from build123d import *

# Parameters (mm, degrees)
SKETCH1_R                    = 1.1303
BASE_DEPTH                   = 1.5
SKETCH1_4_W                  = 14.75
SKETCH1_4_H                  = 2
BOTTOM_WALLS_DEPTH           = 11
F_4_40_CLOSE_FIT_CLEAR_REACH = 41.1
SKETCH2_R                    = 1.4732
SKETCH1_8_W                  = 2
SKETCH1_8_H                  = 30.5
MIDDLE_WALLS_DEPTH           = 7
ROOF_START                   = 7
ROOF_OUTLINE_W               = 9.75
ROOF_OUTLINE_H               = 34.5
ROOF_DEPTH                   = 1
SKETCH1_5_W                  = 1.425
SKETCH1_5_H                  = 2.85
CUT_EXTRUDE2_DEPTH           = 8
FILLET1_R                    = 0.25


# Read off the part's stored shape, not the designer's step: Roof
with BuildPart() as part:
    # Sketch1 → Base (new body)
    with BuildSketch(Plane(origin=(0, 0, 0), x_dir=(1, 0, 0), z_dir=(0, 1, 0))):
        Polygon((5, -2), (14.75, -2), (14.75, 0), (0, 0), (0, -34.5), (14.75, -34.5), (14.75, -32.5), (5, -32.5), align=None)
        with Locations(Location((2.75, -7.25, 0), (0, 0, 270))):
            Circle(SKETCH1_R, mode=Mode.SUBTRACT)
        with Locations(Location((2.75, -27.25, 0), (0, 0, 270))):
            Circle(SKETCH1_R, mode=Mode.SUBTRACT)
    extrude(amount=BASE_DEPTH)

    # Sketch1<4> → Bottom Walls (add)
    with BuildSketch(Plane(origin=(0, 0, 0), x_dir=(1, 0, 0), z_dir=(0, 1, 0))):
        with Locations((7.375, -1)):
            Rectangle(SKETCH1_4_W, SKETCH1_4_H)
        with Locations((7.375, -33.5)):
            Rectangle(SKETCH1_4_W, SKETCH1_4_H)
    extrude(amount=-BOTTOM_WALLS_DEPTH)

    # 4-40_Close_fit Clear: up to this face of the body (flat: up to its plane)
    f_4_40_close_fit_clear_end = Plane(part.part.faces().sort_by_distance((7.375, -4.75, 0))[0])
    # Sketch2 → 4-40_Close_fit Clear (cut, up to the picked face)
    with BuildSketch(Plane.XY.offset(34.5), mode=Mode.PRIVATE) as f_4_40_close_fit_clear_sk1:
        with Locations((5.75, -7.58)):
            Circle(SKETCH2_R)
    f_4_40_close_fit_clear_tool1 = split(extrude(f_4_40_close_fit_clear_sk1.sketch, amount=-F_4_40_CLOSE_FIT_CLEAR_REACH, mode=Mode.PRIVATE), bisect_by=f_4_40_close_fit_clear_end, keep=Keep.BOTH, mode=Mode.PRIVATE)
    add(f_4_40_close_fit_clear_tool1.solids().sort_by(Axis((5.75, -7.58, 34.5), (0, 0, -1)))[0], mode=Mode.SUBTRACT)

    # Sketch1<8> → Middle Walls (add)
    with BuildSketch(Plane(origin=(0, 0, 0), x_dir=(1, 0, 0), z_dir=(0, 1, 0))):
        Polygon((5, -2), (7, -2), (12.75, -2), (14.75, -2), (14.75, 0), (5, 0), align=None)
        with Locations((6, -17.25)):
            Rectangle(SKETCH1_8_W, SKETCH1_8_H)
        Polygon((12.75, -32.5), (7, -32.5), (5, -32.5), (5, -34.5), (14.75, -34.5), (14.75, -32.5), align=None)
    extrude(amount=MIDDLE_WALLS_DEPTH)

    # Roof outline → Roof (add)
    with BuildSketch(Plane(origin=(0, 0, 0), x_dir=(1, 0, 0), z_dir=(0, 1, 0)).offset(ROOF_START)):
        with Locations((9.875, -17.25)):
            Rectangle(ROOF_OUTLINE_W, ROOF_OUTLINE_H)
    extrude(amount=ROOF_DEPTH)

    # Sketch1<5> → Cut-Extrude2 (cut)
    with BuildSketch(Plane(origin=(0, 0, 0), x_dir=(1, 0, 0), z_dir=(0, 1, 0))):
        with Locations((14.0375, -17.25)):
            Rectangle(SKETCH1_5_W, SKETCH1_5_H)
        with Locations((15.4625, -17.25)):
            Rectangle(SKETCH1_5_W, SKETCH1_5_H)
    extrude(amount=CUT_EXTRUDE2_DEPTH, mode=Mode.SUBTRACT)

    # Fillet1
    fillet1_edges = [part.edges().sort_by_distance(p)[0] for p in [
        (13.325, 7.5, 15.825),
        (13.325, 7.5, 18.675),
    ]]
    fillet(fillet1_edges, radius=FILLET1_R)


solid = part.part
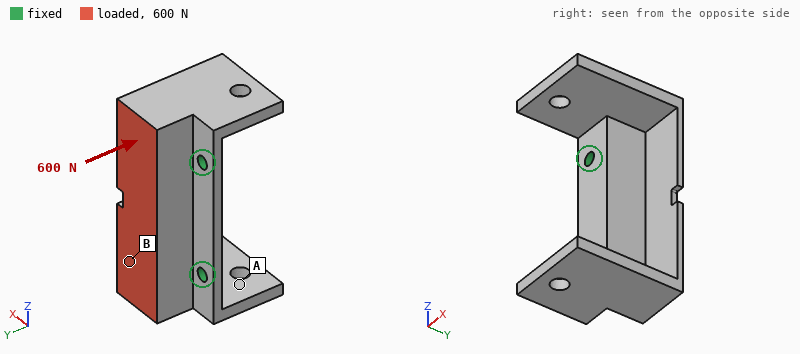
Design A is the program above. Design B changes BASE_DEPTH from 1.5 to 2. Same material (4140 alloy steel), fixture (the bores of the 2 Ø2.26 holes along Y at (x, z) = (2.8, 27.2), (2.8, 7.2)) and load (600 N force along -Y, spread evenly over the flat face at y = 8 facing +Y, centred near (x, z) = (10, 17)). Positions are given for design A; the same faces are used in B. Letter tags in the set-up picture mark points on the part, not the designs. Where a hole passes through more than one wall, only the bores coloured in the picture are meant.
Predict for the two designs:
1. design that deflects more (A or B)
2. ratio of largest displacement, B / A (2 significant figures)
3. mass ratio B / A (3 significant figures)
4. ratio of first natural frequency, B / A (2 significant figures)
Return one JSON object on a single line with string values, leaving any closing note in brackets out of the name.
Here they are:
{"design that deflects more": "A", "ratio of largest displacement, B / A": "0.72", "mass ratio B / A": "1.04", "ratio of first natural frequency, B / A": "1.3"}
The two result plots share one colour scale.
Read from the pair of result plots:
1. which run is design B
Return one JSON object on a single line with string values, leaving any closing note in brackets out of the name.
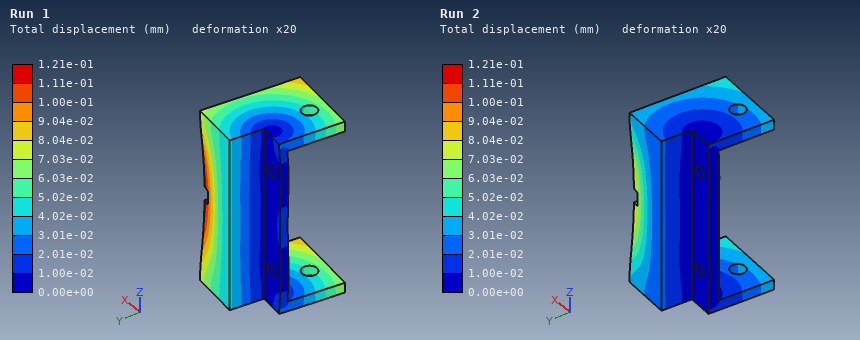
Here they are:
{"which run is design B": "Run 2"}
